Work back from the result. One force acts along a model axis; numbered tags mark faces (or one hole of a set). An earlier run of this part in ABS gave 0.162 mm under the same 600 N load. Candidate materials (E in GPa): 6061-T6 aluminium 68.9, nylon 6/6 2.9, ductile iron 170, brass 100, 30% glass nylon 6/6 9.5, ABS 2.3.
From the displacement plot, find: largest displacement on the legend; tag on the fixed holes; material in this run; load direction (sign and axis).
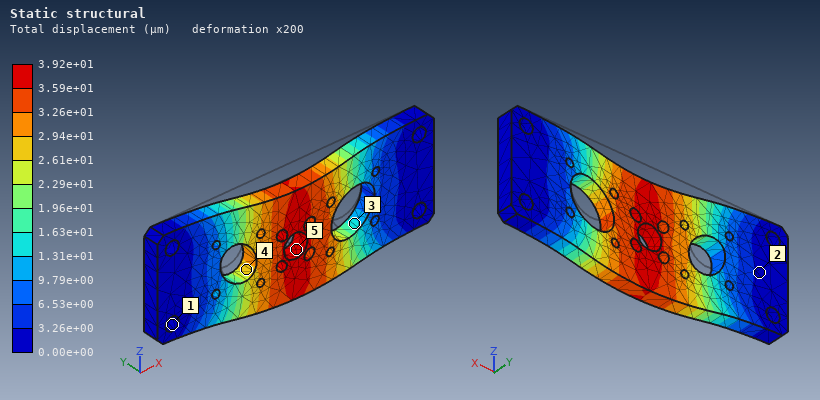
3.92e+01 µm
1
30% glass nylon 6/6
-Z
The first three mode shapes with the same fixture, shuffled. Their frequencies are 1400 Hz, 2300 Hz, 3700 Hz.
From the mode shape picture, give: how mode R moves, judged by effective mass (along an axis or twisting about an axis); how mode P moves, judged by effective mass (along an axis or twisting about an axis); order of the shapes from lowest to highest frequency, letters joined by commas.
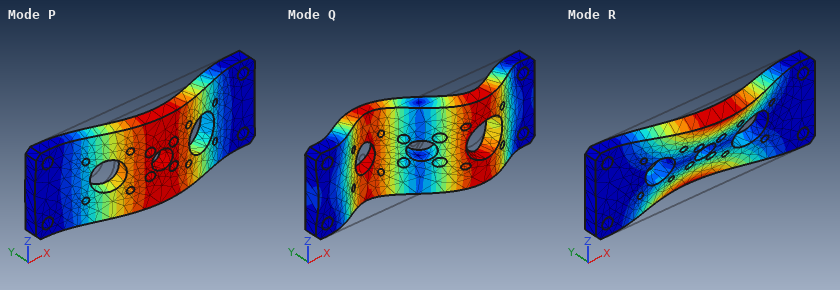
twisting about X
along Y
P, R, Q
